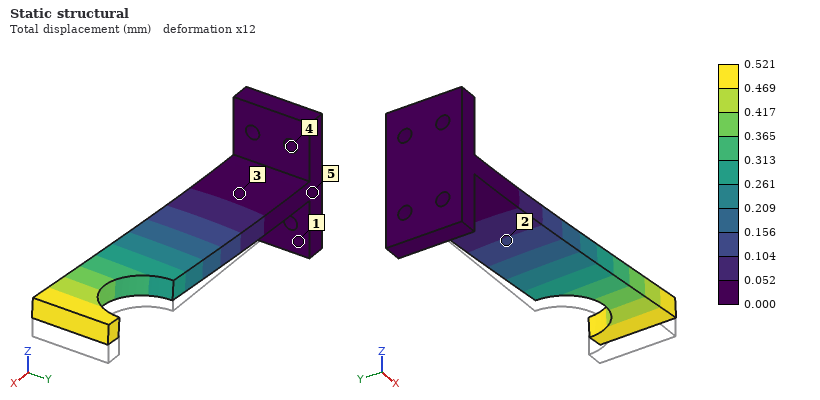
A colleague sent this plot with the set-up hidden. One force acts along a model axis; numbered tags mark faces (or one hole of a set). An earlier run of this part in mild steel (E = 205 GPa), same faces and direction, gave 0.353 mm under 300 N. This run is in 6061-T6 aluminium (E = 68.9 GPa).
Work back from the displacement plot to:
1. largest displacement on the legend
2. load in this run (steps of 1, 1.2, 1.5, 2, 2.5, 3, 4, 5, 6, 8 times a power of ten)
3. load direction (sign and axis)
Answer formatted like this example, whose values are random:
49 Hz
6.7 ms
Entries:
0.521 mm
150 N
+Z
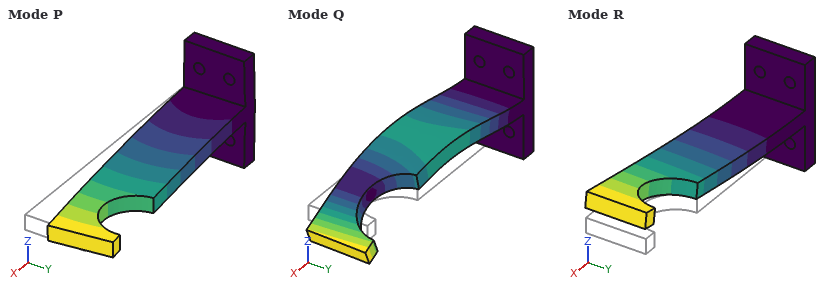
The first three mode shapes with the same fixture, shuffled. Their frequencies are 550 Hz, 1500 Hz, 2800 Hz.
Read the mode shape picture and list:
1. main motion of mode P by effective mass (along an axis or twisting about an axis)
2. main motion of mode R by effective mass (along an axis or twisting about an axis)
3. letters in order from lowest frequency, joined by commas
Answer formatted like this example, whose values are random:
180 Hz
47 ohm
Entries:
along Y
along Z
R, P, Q
